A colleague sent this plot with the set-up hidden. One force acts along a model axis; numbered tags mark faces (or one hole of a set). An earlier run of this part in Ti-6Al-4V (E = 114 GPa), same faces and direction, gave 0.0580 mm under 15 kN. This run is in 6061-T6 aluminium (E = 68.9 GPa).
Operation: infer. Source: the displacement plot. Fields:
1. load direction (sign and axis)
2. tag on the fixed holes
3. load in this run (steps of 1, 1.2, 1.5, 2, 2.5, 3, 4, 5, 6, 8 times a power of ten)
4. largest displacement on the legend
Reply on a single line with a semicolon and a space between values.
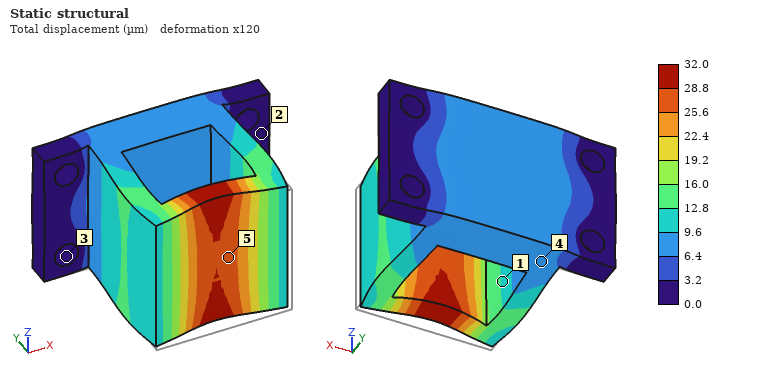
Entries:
+Y; 3; 5 kN; 32.0 µm
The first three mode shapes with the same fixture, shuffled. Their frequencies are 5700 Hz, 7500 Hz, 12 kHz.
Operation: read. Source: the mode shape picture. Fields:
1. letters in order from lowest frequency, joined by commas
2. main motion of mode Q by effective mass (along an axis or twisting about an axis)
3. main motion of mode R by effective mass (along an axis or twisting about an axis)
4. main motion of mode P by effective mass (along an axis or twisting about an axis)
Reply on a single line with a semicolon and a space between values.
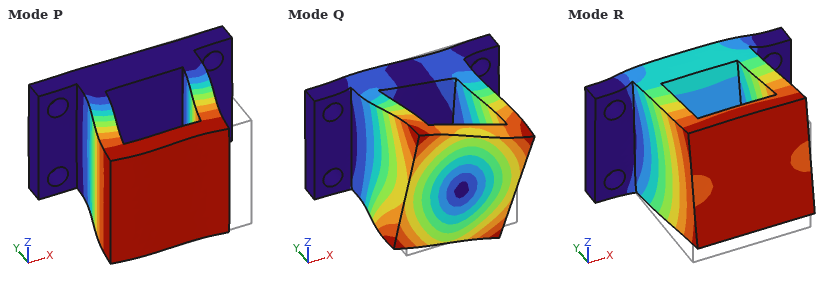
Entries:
P, R, Q; twisting about Y; along Z; along X
